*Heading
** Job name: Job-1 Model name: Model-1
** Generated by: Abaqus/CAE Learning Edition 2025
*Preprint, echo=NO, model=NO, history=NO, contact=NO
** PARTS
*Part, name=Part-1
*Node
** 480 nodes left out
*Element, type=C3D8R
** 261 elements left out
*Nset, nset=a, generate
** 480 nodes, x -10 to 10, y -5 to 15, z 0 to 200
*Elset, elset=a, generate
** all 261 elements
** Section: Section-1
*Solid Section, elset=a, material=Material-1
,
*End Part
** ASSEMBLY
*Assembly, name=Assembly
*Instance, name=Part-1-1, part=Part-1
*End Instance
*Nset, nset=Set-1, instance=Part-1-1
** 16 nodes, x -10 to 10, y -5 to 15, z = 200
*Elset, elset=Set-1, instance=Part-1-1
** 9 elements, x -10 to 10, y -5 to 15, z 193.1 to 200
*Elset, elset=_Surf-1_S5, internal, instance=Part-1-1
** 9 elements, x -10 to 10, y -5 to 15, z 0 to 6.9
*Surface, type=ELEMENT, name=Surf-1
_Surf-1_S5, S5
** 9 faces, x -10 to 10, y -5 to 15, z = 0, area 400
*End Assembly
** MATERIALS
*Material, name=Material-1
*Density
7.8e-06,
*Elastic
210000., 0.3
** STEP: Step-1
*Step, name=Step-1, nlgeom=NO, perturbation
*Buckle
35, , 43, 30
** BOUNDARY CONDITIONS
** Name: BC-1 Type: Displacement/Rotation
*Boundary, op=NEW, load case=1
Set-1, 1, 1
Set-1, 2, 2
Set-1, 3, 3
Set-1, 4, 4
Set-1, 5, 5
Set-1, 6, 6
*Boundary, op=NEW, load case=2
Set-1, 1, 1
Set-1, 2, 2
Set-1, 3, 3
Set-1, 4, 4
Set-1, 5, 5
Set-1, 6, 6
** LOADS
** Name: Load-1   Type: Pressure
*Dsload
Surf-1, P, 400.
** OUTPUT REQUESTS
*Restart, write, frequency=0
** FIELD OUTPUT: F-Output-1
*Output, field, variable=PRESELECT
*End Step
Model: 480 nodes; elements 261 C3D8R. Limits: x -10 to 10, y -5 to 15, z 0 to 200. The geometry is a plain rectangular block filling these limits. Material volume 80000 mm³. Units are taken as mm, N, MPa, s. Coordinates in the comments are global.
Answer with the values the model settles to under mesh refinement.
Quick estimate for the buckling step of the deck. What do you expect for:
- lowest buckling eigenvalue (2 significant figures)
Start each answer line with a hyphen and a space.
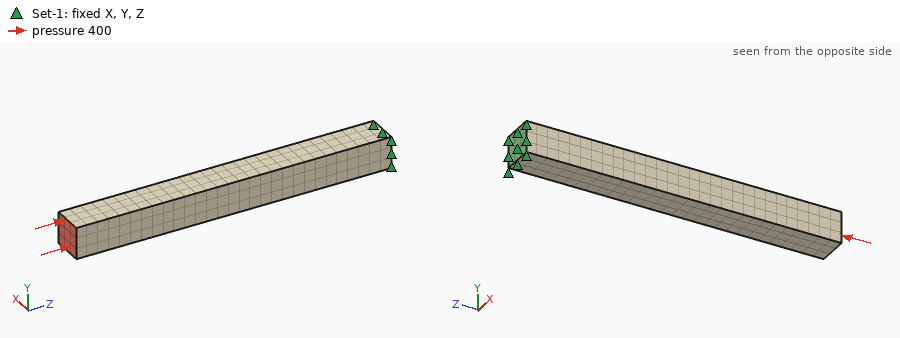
- 1.1
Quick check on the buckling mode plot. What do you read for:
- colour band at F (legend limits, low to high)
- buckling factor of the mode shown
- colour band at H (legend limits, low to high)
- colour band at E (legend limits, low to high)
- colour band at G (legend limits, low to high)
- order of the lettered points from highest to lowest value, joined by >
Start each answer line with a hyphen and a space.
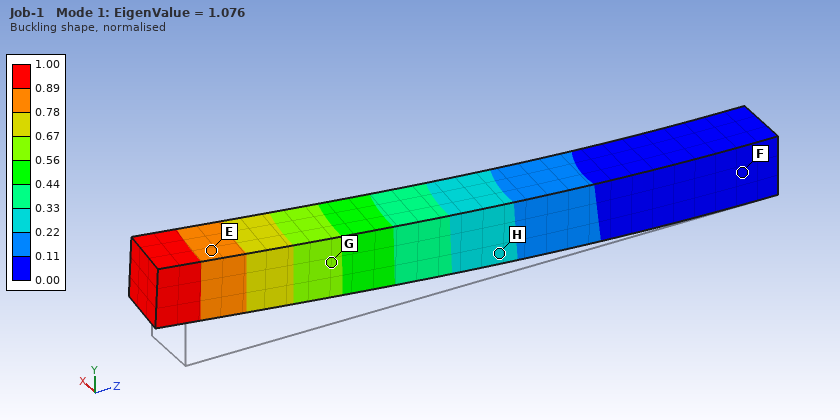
- 0.00 to 0.11
- 1.076
- 0.22 to 0.33
- 0.78 to 0.89
- 0.56 to 0.67
- E > G > H > F
